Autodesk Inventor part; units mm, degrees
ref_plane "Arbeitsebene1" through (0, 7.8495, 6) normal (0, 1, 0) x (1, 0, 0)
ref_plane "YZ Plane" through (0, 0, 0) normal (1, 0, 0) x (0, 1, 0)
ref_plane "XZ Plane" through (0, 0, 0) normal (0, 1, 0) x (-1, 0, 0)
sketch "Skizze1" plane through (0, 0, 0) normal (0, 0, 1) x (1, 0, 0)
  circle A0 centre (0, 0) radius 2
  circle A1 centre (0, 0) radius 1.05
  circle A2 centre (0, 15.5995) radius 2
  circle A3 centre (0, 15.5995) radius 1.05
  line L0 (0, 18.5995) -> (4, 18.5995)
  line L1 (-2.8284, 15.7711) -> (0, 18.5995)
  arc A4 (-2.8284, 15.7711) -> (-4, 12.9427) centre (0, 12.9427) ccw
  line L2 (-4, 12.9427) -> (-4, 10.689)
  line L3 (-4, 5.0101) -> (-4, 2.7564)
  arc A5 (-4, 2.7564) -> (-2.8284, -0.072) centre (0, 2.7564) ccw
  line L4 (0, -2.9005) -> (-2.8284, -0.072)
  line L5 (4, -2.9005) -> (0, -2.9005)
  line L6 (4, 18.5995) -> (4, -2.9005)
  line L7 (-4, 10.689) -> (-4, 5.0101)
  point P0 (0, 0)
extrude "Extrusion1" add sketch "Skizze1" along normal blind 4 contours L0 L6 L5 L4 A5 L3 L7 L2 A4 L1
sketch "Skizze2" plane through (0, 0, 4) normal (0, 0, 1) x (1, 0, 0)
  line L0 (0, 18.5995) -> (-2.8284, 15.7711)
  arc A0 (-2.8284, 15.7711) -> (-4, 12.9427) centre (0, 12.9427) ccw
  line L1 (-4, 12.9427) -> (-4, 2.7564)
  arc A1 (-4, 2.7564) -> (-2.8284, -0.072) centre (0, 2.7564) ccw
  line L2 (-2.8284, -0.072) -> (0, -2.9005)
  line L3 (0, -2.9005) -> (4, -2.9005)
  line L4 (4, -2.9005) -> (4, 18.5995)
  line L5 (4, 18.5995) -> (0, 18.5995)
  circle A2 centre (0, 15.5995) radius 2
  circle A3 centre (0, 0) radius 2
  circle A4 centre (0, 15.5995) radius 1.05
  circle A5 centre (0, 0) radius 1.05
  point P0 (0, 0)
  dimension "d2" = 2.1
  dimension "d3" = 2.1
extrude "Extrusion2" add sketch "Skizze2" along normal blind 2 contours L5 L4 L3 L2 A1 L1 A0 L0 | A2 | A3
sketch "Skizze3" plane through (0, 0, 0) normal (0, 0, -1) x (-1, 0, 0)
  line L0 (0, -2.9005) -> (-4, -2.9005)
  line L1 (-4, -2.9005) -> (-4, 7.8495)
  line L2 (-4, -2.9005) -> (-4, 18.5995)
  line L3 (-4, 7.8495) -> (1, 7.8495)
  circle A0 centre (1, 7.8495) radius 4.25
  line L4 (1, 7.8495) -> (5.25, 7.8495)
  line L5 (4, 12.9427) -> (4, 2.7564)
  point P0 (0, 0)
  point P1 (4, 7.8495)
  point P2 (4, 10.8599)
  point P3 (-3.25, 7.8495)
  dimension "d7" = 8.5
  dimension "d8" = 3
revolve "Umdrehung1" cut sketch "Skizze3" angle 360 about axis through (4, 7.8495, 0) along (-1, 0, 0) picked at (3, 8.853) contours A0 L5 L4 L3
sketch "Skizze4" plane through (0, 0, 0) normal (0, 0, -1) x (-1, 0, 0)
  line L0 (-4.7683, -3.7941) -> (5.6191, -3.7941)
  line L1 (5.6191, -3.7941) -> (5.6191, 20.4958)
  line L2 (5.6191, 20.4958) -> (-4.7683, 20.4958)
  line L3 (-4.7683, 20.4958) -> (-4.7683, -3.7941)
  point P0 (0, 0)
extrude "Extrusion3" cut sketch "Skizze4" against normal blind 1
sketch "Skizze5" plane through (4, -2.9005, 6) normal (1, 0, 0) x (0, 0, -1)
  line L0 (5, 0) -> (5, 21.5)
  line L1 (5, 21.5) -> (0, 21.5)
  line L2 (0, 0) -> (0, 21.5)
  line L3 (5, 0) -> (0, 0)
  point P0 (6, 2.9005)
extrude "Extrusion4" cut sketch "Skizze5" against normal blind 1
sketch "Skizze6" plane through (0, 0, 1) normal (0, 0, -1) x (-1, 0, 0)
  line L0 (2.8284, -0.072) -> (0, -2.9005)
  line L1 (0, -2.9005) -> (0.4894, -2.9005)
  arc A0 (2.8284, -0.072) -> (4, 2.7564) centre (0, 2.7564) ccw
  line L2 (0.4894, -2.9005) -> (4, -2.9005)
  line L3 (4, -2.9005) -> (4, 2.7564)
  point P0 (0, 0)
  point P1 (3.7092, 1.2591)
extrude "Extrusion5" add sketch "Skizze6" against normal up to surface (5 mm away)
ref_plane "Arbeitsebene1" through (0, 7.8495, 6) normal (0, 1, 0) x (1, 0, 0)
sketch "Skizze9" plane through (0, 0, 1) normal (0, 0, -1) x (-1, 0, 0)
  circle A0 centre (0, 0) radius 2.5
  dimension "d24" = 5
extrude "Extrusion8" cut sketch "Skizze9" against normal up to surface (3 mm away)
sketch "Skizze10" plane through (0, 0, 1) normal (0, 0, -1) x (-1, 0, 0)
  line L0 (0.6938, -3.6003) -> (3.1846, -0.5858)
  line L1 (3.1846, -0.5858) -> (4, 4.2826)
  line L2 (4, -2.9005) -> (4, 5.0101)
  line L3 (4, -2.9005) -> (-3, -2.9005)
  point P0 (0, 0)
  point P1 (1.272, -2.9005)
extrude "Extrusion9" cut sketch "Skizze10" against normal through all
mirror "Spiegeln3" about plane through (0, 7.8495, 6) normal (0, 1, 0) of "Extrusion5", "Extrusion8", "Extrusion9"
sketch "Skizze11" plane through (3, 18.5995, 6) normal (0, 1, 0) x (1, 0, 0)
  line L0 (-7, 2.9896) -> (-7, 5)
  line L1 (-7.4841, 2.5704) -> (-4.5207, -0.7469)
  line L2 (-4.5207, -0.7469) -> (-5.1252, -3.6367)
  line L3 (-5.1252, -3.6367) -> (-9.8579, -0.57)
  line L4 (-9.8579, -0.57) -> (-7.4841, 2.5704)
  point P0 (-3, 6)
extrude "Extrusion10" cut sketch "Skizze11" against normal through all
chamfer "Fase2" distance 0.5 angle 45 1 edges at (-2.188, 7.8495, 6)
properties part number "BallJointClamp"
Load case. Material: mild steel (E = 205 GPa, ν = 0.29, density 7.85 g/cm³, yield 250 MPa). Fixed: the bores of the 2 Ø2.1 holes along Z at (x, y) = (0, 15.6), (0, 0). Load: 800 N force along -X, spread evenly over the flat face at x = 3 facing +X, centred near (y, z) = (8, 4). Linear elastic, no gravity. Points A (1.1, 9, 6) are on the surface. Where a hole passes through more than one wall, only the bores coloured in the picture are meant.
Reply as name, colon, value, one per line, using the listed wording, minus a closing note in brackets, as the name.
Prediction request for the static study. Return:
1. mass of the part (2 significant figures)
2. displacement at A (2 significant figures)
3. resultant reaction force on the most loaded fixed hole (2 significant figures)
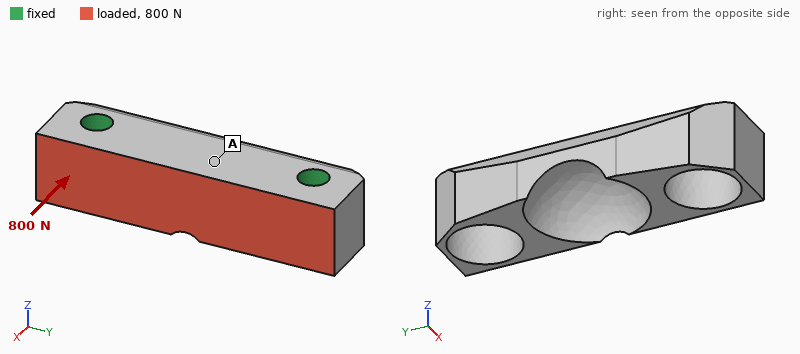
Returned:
mass of the part: 3.4 g
displacement at A: 1.3 µm
resultant reaction force on the most loaded fixed hole: 400 N
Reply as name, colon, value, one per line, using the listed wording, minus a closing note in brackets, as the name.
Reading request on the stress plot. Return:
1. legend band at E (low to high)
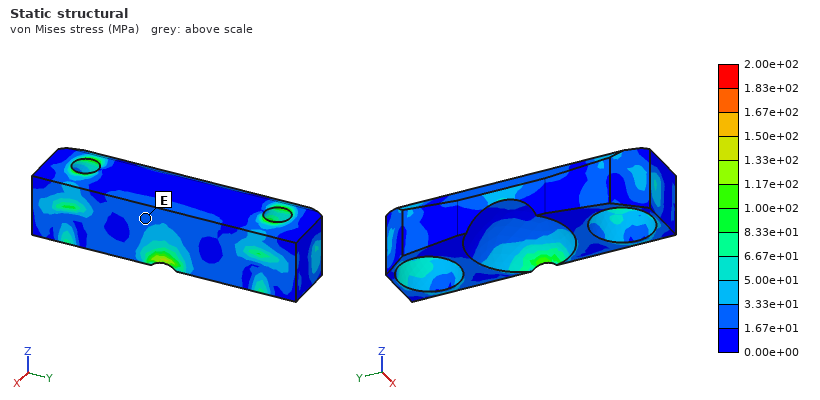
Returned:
legend band at E: 1.67e+01 to 3.33e+01 MPa
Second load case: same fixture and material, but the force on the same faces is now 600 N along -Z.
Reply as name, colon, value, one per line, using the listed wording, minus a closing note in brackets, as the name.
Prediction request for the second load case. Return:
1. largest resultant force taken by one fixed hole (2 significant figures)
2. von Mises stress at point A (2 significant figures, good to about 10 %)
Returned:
largest resultant force taken by one fixed hole: 310 N
von Mises stress at point A: 38 MPa
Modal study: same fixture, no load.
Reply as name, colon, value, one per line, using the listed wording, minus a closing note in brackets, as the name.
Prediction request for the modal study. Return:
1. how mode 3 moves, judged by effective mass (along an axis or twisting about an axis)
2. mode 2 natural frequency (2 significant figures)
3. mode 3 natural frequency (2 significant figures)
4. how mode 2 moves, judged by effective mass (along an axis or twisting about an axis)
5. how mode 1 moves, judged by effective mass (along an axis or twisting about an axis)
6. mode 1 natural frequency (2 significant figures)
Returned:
how mode 3 moves, judged by effective mass: along X
mode 2 natural frequency: 45 kHz
mode 3 natural frequency: 66 kHz
how mode 2 moves, judged by effective mass: along X
how mode 1 moves, judged by effective mass: along Z
mode 1 natural frequency: 42 kHz
